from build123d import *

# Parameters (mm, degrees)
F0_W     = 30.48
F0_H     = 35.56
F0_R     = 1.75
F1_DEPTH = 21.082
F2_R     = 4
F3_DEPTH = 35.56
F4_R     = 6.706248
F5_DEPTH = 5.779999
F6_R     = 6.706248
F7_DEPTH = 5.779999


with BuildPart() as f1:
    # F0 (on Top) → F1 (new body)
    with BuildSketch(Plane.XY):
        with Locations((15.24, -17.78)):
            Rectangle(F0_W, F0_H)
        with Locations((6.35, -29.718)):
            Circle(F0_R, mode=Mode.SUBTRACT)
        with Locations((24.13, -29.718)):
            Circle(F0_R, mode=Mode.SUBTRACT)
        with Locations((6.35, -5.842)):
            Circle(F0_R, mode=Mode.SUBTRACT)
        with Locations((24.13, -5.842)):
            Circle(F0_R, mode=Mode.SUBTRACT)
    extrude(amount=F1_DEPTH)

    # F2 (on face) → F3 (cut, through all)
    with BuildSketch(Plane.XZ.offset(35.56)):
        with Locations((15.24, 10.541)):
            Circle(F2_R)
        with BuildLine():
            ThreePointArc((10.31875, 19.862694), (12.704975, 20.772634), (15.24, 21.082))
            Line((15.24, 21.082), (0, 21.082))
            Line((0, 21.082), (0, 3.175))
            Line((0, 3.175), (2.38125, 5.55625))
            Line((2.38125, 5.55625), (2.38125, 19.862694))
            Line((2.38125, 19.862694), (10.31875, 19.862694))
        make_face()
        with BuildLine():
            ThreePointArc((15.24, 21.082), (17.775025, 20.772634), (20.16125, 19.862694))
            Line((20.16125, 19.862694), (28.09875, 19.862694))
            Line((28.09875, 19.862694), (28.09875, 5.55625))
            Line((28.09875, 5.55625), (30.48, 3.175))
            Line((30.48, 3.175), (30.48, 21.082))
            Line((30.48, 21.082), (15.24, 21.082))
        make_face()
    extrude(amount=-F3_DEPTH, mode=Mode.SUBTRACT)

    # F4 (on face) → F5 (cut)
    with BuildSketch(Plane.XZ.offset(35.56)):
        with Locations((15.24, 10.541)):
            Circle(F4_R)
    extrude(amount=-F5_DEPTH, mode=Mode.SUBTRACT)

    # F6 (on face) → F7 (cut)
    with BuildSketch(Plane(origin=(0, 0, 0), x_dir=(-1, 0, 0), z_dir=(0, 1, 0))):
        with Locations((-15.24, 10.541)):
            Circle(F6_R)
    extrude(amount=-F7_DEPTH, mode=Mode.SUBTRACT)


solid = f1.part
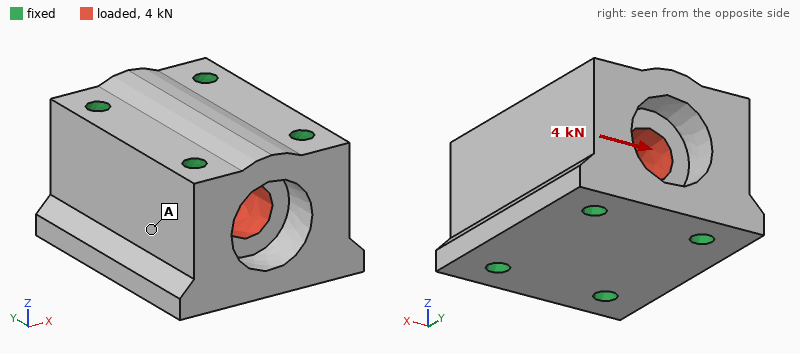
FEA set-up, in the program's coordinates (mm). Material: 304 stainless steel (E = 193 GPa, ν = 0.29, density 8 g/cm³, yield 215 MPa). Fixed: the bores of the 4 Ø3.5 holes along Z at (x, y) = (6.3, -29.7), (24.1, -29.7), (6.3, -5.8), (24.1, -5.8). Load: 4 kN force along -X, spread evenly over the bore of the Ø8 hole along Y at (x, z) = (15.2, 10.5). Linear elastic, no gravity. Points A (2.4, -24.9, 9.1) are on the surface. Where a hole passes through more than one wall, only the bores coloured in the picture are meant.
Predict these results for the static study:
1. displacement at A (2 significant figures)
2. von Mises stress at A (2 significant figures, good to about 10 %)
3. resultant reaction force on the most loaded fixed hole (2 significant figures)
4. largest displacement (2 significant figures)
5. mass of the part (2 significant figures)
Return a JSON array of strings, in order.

["0.27 µm", "2.1 MPa", "1.1 kN", "0.59 µm", "120 g"]
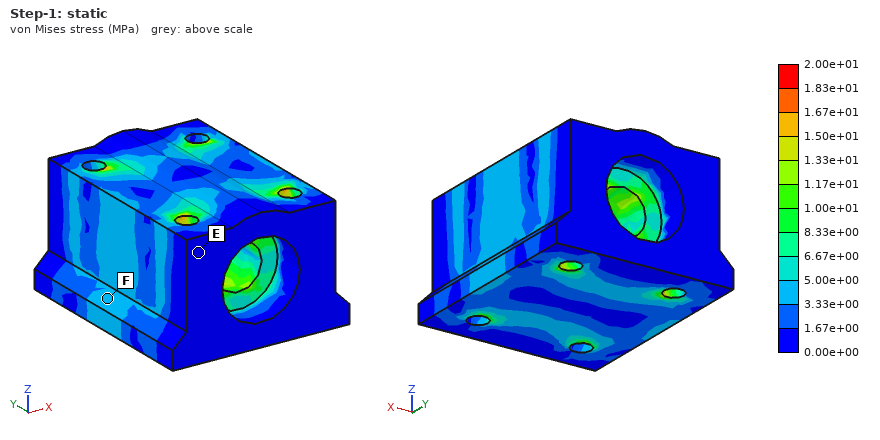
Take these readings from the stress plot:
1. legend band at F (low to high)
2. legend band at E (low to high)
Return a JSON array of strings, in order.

["3.33e+00 to 5.00e+00 MPa", "0.00e+00 to 1.67e+00 MPa"]
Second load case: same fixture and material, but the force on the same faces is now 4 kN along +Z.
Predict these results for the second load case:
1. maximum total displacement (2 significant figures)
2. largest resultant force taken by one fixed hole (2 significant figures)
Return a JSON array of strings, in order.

["0.84 µm", "1.0 kN"]
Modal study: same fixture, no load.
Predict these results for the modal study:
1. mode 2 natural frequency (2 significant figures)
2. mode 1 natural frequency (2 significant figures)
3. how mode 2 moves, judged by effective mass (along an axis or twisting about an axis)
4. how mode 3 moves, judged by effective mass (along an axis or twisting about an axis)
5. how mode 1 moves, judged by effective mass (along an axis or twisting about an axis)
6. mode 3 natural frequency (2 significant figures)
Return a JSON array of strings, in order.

["56 kHz", "53 kHz", "along X", "twisting about Y", "along Z", "60 kHz"]
